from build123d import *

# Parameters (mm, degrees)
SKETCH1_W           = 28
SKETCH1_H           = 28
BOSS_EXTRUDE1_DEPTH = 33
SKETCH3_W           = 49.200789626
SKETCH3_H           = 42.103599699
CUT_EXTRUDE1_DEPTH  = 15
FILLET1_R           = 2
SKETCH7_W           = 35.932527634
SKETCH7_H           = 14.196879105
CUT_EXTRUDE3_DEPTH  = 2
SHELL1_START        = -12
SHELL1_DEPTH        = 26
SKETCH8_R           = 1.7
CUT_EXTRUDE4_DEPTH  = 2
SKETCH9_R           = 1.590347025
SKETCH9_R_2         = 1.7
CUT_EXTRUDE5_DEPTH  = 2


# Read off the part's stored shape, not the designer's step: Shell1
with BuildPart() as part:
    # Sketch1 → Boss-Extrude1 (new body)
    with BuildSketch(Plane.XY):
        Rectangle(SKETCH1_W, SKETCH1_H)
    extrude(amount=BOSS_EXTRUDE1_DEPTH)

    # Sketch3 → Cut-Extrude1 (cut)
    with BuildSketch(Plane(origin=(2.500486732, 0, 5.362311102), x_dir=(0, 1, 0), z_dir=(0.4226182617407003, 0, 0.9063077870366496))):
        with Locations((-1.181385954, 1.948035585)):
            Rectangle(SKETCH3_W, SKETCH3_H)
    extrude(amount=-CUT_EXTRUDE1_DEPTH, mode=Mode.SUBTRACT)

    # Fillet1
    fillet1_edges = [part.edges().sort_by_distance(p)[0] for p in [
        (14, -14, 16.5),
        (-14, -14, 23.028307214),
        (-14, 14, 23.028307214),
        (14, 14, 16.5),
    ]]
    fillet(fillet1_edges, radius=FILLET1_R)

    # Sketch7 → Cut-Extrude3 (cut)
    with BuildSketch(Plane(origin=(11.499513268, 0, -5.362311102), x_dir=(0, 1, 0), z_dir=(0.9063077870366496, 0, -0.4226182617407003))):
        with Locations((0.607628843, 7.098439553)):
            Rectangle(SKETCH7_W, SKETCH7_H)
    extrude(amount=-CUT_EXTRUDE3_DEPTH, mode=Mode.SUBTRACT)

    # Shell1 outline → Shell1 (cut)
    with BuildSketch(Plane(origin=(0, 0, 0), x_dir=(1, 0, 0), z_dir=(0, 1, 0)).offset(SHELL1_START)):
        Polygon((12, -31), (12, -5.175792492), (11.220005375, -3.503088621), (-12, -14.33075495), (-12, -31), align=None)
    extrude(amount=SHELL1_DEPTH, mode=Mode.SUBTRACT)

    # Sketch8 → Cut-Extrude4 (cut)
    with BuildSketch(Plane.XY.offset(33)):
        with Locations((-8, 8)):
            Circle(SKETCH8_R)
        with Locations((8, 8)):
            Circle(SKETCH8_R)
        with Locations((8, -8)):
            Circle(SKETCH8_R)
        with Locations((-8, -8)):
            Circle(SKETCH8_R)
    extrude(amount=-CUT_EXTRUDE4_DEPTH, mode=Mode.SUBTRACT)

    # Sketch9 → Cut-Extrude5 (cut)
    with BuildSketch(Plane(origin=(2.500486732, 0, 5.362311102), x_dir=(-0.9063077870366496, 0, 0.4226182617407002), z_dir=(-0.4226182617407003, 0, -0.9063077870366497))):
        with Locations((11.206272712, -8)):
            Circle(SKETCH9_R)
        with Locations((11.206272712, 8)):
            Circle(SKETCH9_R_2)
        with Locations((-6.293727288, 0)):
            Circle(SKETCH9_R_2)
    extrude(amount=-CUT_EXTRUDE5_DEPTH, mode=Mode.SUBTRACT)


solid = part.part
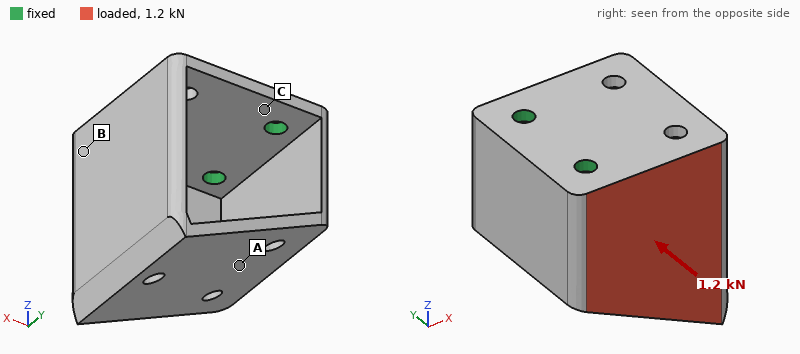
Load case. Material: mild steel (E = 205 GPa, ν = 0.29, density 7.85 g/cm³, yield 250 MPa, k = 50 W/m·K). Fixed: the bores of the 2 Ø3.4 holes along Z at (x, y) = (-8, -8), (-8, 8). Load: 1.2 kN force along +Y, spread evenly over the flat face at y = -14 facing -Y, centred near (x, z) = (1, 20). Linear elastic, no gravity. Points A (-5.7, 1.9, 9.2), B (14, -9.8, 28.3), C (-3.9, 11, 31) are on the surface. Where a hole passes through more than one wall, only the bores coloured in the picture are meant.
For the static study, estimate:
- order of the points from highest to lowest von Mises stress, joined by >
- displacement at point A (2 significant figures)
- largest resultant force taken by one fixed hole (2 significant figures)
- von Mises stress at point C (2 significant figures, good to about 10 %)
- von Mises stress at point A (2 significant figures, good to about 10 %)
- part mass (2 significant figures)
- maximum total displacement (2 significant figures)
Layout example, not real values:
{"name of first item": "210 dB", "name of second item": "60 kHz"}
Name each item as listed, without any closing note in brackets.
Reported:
{"order of the points from highest to lowest von Mises stress, joined by >": "C > A > B", "displacement at point A": "0.053 mm", "largest resultant force taken by one fixed hole": "1.1 kN", "von Mises stress at point C": "92 MPa", "von Mises stress at point A": "50 MPa", "part mass": "51 g", "maximum total displacement": "0.13 mm"}
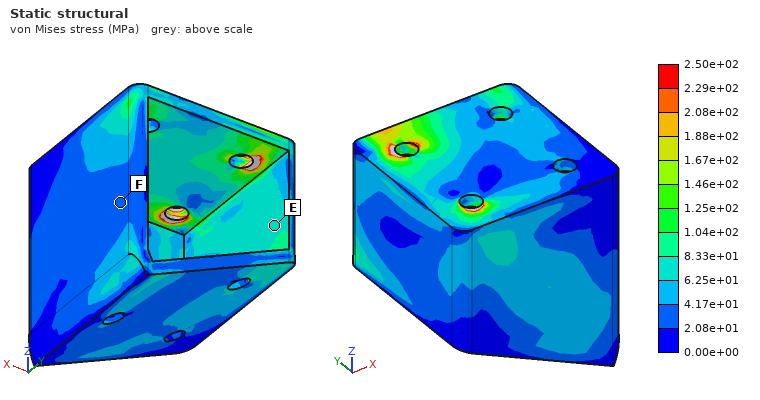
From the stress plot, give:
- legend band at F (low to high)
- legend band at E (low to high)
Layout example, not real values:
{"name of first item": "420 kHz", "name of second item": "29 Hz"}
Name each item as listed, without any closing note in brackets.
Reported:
{"legend band at F": "2.08e+01 to 4.17e+01 MPa", "legend band at E": "6.25e+01 to 8.33e+01 MPa"}
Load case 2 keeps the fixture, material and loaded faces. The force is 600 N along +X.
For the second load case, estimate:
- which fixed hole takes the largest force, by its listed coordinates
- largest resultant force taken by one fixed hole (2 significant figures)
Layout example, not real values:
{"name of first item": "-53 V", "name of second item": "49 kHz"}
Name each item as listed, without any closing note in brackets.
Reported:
{"which fixed hole takes the largest force, by its listed coordinates": "(-8, -8)", "largest resultant force taken by one fixed hole": "740 N"}
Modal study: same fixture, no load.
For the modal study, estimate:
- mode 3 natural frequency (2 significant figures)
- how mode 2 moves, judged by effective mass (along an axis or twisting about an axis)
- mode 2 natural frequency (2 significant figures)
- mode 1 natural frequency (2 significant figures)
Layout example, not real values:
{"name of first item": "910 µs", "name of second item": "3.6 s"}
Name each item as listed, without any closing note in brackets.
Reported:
{"mode 3 natural frequency": "7000 Hz", "how mode 2 moves, judged by effective mass": "along Y", "mode 2 natural frequency": "2400 Hz", "mode 1 natural frequency": "1500 Hz"}
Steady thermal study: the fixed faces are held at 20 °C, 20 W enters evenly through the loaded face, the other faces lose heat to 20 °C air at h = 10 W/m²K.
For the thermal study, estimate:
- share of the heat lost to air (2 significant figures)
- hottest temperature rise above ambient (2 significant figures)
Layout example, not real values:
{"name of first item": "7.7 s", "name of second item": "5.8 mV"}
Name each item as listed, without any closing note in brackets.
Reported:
{"share of the heat lost to air": "14 %", "hottest temperature rise above ambient": "75 K"}
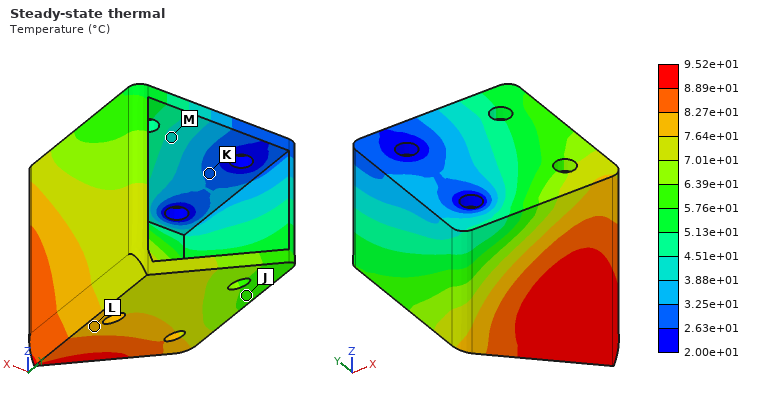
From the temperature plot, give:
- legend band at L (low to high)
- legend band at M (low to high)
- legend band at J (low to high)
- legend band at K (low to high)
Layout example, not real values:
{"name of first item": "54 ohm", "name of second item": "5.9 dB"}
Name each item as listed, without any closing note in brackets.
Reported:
{"legend band at L": "7.64e+01 to 8.27e+01 °C", "legend band at M": "3.88e+01 to 4.51e+01 °C", "legend band at J": "5.76e+01 to 6.39e+01 °C", "legend band at K": "2.63e+01 to 3.25e+01 °C"}
